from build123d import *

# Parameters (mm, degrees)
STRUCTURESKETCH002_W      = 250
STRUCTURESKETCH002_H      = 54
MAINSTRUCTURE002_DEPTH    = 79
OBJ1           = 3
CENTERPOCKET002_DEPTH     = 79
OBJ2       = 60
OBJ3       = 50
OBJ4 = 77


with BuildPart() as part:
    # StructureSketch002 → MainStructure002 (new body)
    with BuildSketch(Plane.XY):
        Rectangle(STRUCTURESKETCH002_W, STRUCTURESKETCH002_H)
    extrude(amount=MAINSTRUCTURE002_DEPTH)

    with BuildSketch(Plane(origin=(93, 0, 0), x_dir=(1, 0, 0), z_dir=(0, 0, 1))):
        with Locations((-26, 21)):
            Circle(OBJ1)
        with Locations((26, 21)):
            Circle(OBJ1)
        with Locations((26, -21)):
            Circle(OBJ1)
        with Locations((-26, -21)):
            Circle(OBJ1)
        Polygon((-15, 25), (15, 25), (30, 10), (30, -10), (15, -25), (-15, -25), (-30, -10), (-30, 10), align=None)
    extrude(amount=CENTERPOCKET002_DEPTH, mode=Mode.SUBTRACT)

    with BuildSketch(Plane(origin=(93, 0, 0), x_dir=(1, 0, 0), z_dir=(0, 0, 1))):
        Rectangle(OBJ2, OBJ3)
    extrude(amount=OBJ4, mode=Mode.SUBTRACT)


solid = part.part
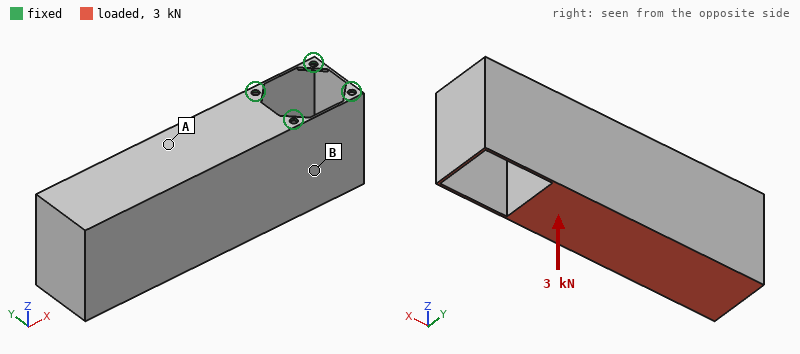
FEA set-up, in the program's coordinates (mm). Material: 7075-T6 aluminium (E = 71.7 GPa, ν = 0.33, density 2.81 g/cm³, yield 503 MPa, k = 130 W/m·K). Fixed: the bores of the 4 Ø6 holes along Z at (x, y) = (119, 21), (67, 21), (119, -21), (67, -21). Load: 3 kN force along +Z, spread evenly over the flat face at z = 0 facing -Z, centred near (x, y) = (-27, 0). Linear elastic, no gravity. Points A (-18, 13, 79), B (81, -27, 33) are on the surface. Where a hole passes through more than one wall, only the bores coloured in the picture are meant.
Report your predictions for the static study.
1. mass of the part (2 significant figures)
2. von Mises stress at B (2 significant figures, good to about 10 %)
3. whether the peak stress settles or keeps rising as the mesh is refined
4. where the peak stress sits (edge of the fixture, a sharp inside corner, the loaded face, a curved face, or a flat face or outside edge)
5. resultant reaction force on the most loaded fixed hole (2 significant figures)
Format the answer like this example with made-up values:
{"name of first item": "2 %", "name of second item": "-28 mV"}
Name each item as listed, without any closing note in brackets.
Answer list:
{"mass of the part": "2.3 kg", "von Mises stress at B": "32 MPa", "whether the peak stress settles or keeps rising as the mesh is refined": "keeps rising", "where the peak stress sits": "edge of the fixture", "resultant reaction force on the most loaded fixed hole": "4.1 kN"}
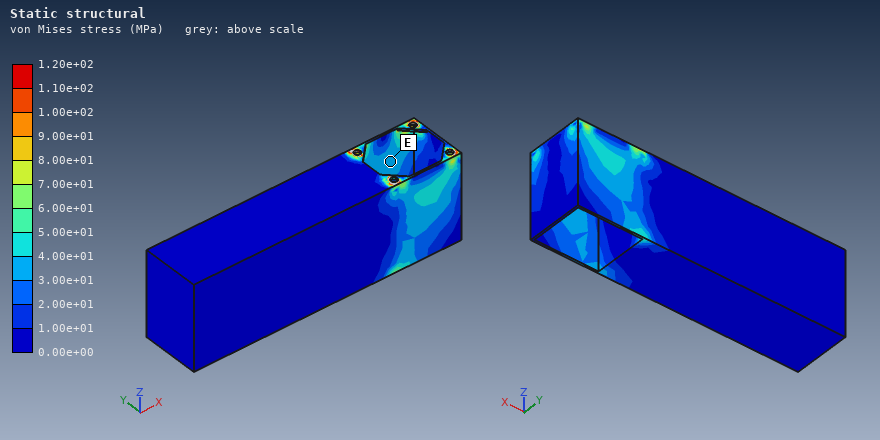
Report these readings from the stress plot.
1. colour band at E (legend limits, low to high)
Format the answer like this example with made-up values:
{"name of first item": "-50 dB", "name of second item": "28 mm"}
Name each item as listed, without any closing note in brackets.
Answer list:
{"colour band at E": "3.00e+01 to 4.00e+01 MPa"}
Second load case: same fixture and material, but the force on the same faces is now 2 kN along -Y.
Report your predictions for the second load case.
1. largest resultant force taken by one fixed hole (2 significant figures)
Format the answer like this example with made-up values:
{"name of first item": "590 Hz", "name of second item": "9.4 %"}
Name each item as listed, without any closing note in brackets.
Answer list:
{"largest resultant force taken by one fixed hole": "4.5 kN"}
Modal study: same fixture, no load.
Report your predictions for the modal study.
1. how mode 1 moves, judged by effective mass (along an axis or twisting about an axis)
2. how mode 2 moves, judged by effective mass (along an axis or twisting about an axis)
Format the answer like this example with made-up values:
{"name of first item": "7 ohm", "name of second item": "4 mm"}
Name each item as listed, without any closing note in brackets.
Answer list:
{"how mode 1 moves, judged by effective mass": "along Z", "how mode 2 moves, judged by effective mass": "along Y"}
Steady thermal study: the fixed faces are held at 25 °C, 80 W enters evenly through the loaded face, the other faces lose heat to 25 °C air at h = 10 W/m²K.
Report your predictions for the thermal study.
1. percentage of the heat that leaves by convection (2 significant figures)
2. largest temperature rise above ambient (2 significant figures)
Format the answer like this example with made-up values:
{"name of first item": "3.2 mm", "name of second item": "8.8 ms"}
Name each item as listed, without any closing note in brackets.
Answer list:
{"percentage of the heat that leaves by convection": "28 %", "largest temperature rise above ambient": "43 K"}
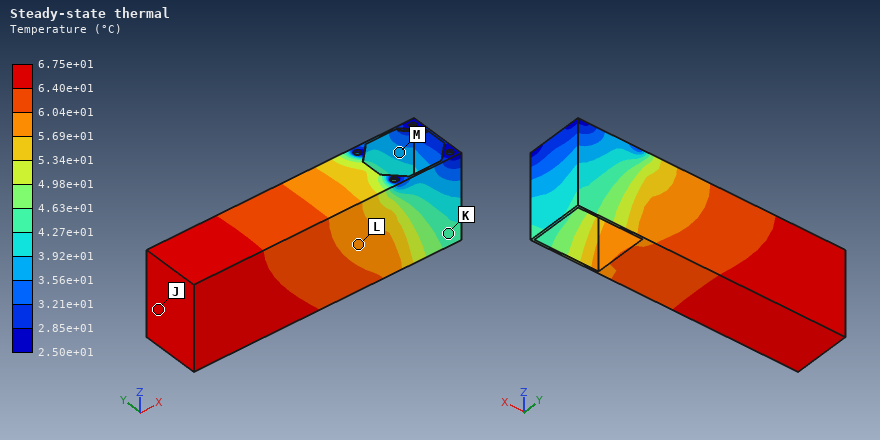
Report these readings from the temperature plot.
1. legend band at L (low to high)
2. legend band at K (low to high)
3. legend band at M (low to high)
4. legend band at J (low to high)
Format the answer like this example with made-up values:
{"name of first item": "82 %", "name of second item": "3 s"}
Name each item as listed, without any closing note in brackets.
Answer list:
{"legend band at L": "5.69e+01 to 6.04e+01 °C", "legend band at K": "4.27e+01 to 4.63e+01 °C", "legend band at M": "3.56e+01 to 3.92e+01 °C", "legend band at J": "6.40e+01 to 6.75e+01 °C"}
